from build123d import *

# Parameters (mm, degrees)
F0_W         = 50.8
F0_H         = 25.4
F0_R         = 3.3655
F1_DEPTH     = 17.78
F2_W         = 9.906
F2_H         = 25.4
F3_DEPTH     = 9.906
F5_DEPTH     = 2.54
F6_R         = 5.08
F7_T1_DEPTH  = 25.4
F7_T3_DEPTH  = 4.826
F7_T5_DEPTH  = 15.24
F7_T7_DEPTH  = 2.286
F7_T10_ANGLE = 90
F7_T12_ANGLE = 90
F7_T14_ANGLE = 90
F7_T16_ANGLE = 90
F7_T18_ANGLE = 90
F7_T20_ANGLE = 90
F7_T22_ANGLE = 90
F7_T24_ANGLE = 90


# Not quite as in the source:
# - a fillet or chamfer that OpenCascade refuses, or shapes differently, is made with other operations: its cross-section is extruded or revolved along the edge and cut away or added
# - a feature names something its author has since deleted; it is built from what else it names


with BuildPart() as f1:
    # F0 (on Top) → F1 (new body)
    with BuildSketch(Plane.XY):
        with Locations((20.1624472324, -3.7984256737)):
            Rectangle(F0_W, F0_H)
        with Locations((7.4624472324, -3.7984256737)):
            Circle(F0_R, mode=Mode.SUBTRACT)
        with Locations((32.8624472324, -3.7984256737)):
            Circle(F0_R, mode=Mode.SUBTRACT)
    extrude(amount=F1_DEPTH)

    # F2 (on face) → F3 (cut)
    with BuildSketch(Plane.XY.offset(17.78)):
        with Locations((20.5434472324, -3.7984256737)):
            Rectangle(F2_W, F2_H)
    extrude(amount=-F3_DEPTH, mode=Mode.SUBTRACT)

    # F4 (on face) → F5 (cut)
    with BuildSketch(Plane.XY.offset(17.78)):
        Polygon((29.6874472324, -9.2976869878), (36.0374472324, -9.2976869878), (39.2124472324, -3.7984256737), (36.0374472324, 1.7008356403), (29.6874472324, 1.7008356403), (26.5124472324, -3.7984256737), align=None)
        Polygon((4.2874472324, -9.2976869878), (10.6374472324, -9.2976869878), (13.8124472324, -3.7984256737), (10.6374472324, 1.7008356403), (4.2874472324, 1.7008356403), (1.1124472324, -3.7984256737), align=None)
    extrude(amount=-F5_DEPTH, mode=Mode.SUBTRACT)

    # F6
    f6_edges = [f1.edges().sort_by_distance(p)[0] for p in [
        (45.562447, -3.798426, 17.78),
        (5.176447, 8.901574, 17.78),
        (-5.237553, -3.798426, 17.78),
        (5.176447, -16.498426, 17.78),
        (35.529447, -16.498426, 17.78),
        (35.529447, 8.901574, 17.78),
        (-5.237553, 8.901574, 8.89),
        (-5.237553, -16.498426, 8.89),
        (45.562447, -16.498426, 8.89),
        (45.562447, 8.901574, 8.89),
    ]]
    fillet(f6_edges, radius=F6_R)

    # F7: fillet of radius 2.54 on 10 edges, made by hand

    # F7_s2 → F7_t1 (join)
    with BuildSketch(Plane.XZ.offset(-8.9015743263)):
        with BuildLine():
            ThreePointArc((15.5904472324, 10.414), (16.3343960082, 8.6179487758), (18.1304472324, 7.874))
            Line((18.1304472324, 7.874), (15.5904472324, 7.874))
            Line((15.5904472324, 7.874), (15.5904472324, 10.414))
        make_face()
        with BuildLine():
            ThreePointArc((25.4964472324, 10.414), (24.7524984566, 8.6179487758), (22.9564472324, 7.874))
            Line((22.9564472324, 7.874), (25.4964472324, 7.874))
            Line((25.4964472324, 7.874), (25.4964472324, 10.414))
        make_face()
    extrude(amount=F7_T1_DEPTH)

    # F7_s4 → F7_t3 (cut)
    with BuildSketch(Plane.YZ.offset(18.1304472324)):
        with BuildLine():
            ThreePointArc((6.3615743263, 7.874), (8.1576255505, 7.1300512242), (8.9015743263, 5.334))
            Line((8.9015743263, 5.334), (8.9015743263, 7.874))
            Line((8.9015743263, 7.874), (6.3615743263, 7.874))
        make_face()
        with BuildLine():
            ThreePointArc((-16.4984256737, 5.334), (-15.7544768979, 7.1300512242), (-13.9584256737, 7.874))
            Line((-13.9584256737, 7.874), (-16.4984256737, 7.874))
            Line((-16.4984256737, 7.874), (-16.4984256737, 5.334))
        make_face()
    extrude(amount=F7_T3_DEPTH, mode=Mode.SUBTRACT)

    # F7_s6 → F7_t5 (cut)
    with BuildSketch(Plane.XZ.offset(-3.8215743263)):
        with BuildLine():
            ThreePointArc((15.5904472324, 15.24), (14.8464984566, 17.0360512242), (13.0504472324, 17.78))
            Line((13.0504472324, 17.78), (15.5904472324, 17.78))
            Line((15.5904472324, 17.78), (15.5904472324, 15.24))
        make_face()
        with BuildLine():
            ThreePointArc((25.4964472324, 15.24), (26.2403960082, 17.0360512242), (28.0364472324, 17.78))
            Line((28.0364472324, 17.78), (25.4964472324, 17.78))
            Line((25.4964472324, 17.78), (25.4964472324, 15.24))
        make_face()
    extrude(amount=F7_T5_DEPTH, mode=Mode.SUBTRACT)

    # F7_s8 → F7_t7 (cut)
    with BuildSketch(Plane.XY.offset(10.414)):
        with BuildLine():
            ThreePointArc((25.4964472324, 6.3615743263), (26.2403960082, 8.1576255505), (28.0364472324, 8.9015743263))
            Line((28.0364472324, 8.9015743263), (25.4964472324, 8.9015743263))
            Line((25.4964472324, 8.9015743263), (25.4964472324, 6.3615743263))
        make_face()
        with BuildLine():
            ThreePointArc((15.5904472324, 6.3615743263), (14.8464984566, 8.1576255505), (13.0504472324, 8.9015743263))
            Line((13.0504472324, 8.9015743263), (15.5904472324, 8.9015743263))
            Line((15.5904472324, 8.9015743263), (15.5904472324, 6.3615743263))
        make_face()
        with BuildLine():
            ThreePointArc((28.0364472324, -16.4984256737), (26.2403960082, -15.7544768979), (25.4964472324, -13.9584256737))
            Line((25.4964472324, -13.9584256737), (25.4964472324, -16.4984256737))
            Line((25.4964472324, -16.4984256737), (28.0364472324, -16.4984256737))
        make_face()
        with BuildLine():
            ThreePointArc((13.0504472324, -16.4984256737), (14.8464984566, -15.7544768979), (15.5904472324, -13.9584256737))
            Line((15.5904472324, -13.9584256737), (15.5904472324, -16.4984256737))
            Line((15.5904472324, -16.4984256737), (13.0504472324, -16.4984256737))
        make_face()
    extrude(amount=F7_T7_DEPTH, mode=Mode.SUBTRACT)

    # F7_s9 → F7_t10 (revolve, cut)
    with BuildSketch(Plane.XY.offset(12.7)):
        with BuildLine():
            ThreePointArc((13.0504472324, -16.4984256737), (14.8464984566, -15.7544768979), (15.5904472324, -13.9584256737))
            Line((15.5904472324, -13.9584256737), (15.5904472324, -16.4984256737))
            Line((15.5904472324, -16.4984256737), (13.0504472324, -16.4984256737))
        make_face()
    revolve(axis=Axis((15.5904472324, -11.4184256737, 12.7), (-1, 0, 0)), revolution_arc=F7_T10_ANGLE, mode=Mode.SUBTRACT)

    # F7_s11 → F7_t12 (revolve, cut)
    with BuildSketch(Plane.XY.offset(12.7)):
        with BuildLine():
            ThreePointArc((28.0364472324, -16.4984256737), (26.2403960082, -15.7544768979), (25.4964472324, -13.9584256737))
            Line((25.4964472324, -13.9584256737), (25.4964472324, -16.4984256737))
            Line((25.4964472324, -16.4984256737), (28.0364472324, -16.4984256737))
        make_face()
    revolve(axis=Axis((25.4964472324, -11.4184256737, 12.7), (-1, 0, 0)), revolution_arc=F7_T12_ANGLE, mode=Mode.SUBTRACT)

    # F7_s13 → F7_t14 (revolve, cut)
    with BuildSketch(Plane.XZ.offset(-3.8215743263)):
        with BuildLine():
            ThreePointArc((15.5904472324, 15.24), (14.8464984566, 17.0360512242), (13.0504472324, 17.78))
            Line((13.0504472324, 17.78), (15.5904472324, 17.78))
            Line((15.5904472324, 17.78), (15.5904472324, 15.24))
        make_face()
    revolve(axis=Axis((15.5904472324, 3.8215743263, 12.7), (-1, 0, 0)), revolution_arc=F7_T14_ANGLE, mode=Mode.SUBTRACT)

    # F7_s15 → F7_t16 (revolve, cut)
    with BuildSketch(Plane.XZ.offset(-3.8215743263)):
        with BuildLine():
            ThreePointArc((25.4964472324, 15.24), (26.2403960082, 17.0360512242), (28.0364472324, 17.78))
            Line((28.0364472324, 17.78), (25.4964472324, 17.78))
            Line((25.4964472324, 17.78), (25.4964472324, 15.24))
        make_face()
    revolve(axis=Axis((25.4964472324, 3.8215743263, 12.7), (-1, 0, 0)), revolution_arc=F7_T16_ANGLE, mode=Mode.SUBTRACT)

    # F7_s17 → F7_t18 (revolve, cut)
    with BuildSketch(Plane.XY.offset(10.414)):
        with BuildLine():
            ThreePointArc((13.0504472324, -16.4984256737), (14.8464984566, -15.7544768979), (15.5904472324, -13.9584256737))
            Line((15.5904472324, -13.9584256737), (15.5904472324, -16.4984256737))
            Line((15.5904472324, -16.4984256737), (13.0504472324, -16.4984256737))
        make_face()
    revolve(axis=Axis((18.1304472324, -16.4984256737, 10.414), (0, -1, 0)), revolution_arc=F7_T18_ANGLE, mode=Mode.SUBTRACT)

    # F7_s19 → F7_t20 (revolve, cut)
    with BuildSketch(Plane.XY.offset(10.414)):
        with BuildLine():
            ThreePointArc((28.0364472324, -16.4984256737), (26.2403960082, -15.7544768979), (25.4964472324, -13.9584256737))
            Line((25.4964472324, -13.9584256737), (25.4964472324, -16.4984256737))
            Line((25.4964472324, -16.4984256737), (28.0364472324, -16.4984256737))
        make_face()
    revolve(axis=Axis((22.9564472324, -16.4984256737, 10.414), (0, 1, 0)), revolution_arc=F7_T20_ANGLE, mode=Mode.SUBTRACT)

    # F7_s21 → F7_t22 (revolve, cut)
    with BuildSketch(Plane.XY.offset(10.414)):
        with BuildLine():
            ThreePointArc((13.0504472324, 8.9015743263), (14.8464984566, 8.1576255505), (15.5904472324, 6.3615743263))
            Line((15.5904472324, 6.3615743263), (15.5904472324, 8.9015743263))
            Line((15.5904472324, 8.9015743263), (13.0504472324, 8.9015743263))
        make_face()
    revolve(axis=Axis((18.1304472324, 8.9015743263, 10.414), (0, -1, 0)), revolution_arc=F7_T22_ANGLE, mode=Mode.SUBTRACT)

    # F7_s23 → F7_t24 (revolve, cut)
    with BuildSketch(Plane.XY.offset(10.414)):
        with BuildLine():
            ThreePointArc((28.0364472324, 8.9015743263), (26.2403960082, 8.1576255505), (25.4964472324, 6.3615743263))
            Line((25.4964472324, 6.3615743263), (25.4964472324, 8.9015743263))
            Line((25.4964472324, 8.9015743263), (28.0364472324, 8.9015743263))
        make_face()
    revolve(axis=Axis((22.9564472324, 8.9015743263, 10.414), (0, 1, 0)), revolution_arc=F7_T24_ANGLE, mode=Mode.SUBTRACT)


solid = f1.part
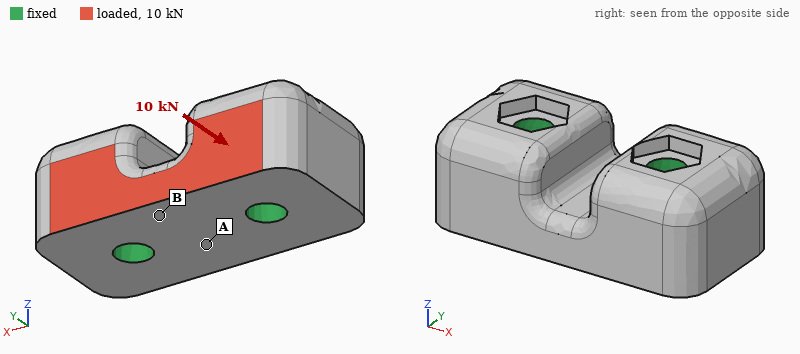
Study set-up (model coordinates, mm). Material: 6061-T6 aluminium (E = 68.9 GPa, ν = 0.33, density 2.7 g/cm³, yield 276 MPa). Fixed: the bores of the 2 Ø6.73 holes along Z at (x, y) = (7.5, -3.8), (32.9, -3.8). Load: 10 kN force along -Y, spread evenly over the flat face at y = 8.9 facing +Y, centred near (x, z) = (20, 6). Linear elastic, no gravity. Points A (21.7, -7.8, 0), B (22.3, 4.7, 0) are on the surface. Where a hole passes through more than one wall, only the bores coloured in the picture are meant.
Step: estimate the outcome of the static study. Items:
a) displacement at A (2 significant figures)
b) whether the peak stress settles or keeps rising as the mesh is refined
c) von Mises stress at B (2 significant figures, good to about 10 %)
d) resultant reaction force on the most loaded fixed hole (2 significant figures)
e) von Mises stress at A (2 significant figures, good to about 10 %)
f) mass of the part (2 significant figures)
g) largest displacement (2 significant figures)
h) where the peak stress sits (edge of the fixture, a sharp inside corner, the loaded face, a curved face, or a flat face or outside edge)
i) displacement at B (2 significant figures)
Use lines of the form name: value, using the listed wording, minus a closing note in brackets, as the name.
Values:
displacement at A: 2.0 µm
whether the peak stress settles or keeps rising as the mesh is refined: keeps rising
von Mises stress at B: 22 MPa
resultant reaction force on the most loaded fixed hole: 5.1 kN
von Mises stress at A: 7.5 MPa
mass of the part: 48 g
largest displacement: 6.8 µm
where the peak stress sits: edge of the fixture
displacement at B: 4.8 µm
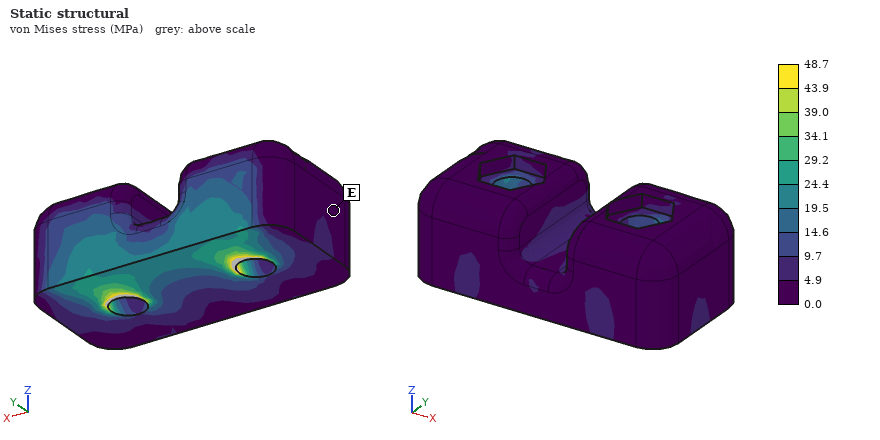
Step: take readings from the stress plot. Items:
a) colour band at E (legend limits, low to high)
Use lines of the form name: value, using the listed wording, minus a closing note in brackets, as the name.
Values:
colour band at E: 0.0 to 4.9 MPa
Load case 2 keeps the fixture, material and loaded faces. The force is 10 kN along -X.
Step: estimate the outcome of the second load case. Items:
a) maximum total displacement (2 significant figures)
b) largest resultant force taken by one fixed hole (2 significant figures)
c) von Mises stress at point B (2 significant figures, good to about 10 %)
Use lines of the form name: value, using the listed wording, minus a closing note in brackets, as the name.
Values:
maximum total displacement: 14 µm
largest resultant force taken by one fixed hole: 5.8 kN
von Mises stress at point B: 42 MPa
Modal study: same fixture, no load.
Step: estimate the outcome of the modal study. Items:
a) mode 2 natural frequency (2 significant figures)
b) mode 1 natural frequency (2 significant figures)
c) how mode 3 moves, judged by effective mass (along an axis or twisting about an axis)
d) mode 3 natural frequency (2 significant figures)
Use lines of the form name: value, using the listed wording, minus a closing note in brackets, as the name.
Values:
mode 2 natural frequency: 36 kHz
mode 1 natural frequency: 35 kHz
how mode 3 moves, judged by effective mass: twisting about X
mode 3 natural frequency: 40 kHz
